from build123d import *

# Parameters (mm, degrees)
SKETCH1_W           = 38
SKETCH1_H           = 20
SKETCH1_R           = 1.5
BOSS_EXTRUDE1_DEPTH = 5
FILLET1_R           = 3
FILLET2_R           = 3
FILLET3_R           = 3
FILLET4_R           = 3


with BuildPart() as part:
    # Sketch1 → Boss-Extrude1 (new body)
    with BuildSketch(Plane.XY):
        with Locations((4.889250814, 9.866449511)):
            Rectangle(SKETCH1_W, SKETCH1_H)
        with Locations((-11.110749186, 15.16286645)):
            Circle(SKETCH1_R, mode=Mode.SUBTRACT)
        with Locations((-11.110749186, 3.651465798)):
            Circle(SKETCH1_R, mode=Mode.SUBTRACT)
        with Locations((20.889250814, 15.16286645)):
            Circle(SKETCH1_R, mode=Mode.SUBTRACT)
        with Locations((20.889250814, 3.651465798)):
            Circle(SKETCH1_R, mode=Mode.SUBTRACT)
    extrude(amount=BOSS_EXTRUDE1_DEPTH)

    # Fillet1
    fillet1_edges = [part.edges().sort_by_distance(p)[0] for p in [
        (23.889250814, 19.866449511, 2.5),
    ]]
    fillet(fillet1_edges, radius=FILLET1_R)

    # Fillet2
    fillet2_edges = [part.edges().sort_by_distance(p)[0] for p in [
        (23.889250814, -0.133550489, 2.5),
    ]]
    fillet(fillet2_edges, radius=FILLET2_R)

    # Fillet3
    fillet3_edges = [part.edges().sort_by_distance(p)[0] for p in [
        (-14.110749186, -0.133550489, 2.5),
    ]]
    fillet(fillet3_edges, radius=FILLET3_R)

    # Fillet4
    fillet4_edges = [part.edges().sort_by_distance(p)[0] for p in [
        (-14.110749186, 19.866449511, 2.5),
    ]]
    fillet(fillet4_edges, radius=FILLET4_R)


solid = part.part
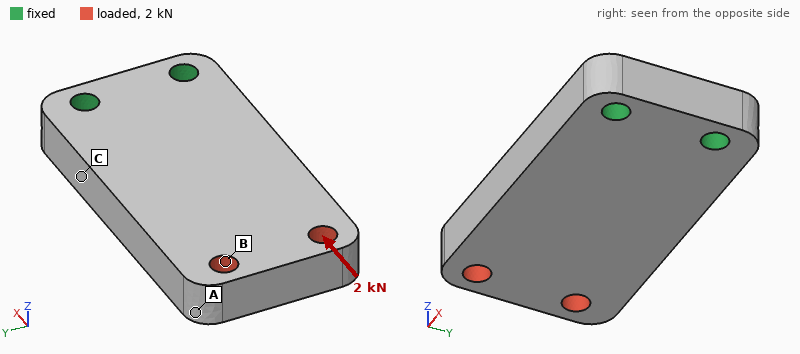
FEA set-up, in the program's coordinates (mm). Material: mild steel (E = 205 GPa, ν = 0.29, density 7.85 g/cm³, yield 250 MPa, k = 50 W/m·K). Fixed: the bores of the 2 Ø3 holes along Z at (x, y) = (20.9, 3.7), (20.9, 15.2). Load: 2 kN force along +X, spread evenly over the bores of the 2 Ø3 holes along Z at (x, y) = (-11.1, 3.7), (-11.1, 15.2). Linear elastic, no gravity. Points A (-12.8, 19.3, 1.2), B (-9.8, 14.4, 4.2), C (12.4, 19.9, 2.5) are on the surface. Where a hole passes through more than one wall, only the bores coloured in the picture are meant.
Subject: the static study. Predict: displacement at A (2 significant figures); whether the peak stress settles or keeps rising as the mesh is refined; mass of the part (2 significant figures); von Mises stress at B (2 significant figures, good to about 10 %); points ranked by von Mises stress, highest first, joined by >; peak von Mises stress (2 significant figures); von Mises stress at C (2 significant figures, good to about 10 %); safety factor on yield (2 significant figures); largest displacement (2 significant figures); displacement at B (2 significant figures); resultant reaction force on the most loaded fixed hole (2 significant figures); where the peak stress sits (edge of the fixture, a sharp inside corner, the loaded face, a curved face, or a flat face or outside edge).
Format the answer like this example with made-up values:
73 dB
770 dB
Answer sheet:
2.8 µm
settles
28 g
31 MPa
B > C > A
72 MPa
16 MPa
3.5
4.4 µm
3.0 µm
1.0 kN
the loaded face
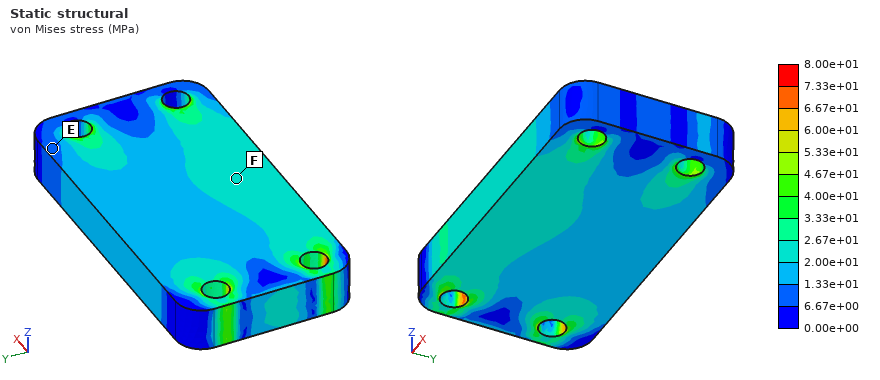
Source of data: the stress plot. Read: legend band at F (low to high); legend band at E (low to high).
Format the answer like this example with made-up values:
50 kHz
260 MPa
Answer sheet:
2.00e+01 to 2.67e+01 MPa
6.67e+00 to 1.33e+01 MPa
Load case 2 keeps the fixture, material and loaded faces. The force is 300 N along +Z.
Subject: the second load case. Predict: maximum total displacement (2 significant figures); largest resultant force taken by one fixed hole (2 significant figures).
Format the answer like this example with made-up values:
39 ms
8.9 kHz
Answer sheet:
88 µm
160 N
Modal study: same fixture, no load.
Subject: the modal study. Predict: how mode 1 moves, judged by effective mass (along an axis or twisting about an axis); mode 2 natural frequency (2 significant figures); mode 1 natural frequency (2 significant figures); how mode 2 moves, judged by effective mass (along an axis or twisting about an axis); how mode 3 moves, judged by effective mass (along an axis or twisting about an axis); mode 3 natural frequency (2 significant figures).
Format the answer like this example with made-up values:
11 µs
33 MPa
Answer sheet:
along Z
11 kHz
3500 Hz
along Y
twisting about X
12 kHz
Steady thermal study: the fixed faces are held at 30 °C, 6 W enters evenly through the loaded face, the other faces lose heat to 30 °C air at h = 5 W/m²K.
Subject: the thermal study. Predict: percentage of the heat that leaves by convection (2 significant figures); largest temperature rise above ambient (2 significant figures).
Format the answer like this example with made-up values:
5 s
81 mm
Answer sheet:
3.1 %
41 K
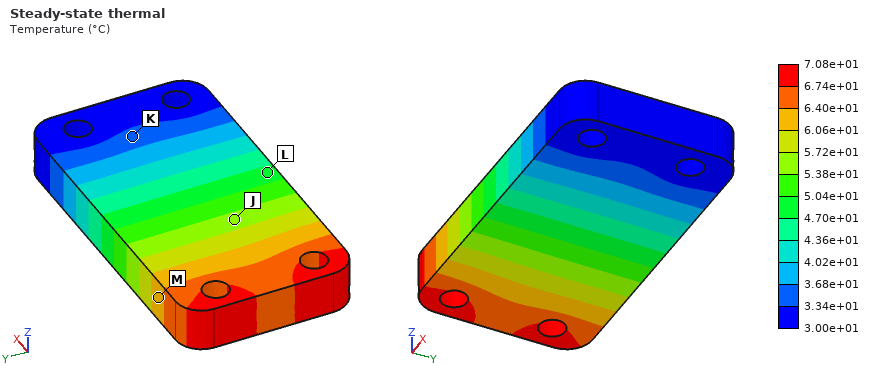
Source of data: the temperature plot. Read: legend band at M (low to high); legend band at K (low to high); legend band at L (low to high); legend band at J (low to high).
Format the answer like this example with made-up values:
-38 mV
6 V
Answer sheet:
6.06e+01 to 6.40e+01 °C
3.34e+01 to 3.68e+01 °C
4.70e+01 to 5.04e+01 °C
5.38e+01 to 5.72e+01 °C
